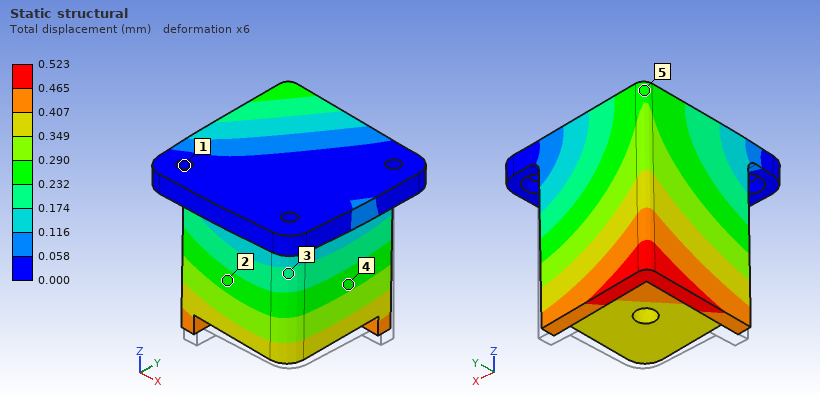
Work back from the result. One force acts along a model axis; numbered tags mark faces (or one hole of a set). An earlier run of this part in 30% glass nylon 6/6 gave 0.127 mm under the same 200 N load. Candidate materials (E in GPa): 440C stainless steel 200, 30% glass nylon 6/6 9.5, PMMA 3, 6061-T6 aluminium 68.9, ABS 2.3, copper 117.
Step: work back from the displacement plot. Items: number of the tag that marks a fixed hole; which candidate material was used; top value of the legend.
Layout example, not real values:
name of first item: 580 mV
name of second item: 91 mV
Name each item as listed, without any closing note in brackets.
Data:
number of the tag that marks a fixed hole: 1
which candidate material was used: ABS
top value of the legend: 0.523 mm
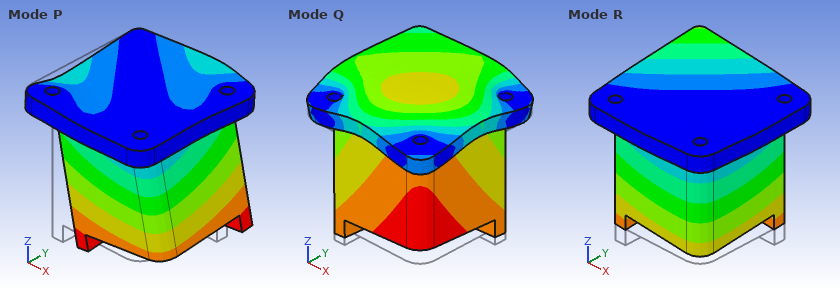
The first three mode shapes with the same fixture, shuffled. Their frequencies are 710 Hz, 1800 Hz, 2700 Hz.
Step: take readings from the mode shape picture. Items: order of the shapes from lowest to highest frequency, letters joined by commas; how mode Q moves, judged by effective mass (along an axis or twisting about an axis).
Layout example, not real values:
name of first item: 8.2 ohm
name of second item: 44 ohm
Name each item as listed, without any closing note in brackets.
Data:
order of the shapes from lowest to highest frequency, letters joined by commas: R, P, Q
how mode Q moves, judged by effective mass: along Z
